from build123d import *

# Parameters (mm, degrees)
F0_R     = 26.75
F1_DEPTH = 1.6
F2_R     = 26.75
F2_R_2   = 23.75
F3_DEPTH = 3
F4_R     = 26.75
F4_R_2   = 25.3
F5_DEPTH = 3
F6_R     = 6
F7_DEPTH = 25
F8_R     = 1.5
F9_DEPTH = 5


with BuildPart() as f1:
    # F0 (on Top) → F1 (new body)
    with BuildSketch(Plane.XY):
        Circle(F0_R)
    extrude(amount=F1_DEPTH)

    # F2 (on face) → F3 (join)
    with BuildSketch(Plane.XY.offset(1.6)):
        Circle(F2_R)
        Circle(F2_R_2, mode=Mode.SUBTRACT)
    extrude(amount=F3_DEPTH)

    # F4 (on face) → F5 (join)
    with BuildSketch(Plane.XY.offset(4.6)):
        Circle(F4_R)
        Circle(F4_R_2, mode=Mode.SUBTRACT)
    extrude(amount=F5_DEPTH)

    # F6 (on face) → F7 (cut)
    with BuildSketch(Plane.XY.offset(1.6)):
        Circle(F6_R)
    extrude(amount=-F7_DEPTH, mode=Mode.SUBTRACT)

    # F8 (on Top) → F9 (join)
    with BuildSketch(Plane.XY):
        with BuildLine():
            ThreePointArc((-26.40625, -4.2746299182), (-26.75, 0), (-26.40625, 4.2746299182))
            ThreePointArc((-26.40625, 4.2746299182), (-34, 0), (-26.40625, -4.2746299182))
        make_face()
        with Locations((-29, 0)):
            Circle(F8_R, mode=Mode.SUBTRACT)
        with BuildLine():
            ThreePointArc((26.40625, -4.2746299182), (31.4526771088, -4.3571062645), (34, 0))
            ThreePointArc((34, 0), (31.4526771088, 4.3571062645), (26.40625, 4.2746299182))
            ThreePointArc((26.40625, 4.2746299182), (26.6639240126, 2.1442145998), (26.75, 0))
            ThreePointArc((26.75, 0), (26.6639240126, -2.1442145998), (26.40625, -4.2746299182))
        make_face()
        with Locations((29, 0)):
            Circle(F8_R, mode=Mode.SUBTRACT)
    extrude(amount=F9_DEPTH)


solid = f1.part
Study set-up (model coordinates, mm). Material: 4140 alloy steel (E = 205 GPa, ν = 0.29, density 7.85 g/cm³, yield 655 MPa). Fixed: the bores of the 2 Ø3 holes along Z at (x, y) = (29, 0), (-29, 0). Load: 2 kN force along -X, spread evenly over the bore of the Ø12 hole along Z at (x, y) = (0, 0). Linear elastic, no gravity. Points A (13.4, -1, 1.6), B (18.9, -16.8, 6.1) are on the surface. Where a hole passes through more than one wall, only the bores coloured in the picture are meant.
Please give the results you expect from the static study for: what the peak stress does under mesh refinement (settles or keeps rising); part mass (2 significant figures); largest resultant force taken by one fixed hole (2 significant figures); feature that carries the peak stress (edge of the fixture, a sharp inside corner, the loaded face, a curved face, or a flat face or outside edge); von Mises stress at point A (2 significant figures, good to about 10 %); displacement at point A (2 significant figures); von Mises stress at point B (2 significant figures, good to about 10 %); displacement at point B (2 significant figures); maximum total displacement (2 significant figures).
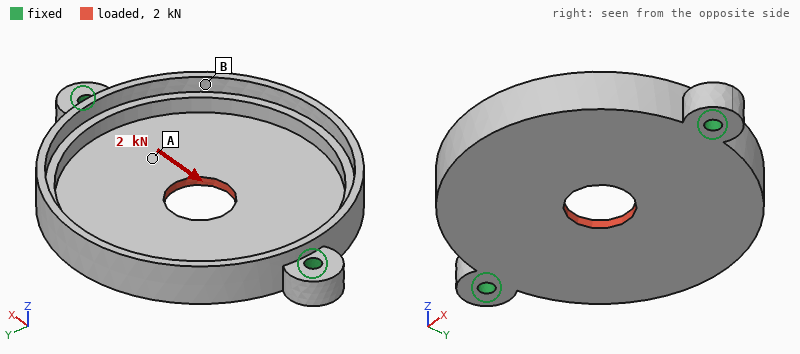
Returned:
keeps rising
48 g
1.0 kN
edge of the fixture
42 MPa
3.7 µm
7.8 MPa
3.6 µm
5.1 µm
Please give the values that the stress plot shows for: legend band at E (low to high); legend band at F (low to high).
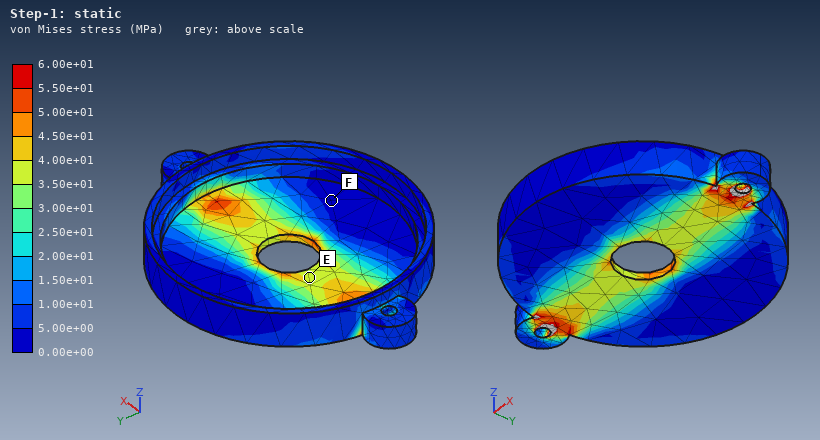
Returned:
3.50e+01 to 4.00e+01 MPa
0.00e+00 to 5.00e+00 MPa
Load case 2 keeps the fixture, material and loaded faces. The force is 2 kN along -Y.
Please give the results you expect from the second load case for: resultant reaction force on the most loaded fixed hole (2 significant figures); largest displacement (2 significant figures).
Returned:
1.0 kN
23 µm
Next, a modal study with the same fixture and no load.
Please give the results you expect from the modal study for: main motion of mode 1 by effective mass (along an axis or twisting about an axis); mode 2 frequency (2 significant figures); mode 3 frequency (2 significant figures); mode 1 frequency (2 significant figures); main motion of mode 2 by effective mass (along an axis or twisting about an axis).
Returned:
twisting about X
4000 Hz
7000 Hz
3300 Hz
along Z
